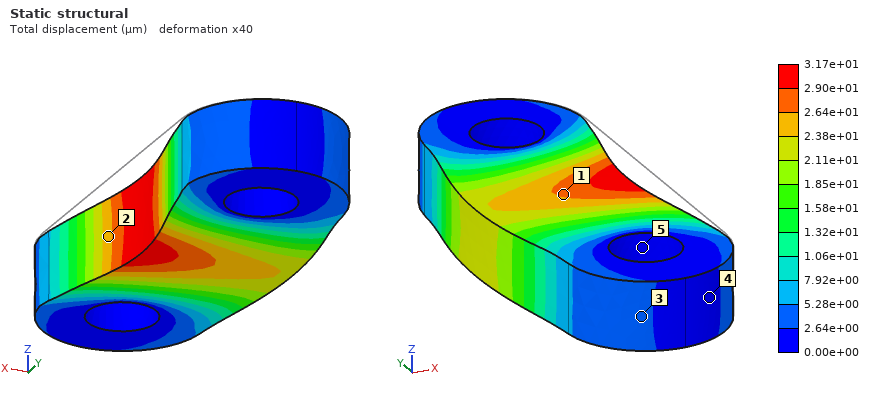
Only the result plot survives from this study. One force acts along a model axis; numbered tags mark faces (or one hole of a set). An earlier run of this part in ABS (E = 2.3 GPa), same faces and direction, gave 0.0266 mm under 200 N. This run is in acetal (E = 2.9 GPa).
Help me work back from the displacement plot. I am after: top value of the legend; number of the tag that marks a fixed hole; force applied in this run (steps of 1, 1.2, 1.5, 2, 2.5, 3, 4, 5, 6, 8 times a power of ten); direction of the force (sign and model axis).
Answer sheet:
3.17e+01 µm
5
300 N
-X
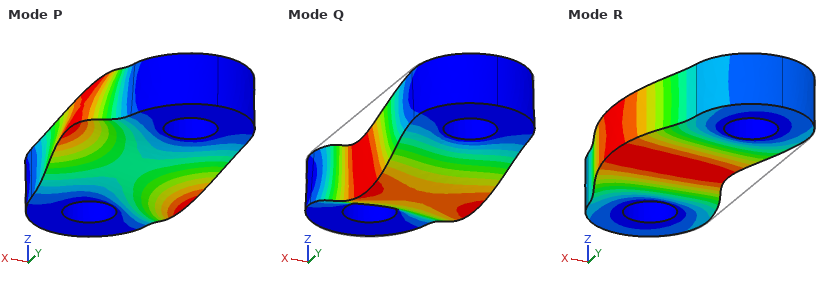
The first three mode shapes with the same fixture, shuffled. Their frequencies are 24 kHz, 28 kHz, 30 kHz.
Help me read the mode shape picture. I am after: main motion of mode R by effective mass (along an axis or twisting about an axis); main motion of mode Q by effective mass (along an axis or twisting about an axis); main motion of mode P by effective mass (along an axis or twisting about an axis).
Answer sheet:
along X
along Z
twisting about Y
